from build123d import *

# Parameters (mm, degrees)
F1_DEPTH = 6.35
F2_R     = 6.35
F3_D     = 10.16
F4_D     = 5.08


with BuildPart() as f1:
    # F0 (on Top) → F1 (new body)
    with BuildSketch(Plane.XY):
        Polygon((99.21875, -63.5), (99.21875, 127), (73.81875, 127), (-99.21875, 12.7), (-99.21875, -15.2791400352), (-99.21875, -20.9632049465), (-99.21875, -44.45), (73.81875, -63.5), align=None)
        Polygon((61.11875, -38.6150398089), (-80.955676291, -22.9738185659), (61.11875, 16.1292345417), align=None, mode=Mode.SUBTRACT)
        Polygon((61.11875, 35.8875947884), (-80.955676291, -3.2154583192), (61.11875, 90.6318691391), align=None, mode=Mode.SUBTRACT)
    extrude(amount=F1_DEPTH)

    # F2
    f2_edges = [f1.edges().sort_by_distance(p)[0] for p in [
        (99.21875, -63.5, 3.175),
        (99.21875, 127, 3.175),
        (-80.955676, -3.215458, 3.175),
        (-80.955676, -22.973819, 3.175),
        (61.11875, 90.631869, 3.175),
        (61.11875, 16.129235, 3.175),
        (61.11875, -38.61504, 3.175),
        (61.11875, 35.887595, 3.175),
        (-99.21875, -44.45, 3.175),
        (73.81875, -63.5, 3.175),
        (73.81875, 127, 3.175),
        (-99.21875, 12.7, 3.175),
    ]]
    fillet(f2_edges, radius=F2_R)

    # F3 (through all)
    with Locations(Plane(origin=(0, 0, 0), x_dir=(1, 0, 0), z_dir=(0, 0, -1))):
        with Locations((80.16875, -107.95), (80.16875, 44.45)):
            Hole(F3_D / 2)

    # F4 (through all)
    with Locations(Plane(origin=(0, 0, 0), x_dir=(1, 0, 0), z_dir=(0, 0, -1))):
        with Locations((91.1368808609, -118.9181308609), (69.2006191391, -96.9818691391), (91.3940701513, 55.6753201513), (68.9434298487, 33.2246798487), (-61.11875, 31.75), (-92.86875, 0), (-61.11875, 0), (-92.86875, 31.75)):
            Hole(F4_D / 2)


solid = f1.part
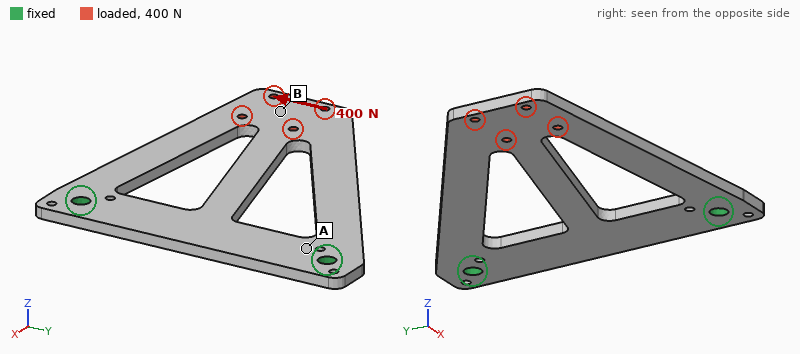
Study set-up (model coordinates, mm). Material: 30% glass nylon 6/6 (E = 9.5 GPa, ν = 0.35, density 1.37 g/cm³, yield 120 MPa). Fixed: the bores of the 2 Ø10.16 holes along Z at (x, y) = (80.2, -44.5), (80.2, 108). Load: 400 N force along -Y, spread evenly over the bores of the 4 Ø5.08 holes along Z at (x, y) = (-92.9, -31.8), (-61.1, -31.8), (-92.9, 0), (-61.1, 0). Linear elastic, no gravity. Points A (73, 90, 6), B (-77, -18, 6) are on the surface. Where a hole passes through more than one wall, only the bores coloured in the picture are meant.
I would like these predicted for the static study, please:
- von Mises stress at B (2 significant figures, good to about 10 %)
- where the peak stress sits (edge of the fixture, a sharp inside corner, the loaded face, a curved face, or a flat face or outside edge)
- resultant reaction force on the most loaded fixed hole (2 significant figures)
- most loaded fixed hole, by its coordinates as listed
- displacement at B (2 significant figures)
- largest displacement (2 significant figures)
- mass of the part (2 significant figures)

1.6 MPa
a curved face
470 N
(80.2, 108)
0.18 mm
0.20 mm
160 g
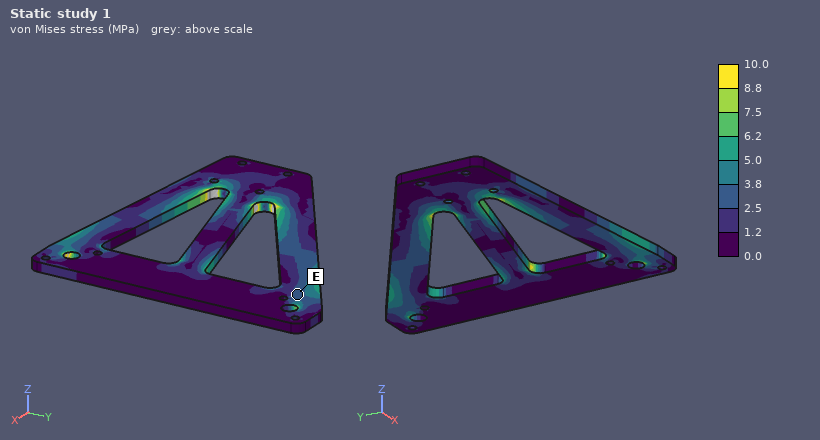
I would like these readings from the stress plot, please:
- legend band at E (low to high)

2.5 to 3.8 MPa
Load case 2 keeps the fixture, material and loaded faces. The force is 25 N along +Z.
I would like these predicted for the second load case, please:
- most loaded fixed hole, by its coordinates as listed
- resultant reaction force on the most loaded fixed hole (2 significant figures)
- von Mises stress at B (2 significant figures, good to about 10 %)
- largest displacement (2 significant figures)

(80.2, -44.5)
19 N
1.3 MPa
3.0 mm
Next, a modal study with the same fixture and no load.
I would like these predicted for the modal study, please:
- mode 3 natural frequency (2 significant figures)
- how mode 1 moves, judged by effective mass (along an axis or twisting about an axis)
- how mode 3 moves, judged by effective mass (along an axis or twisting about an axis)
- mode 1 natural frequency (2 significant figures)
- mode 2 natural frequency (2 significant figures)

490 Hz
along Z
along Z
82 Hz
330 Hz
